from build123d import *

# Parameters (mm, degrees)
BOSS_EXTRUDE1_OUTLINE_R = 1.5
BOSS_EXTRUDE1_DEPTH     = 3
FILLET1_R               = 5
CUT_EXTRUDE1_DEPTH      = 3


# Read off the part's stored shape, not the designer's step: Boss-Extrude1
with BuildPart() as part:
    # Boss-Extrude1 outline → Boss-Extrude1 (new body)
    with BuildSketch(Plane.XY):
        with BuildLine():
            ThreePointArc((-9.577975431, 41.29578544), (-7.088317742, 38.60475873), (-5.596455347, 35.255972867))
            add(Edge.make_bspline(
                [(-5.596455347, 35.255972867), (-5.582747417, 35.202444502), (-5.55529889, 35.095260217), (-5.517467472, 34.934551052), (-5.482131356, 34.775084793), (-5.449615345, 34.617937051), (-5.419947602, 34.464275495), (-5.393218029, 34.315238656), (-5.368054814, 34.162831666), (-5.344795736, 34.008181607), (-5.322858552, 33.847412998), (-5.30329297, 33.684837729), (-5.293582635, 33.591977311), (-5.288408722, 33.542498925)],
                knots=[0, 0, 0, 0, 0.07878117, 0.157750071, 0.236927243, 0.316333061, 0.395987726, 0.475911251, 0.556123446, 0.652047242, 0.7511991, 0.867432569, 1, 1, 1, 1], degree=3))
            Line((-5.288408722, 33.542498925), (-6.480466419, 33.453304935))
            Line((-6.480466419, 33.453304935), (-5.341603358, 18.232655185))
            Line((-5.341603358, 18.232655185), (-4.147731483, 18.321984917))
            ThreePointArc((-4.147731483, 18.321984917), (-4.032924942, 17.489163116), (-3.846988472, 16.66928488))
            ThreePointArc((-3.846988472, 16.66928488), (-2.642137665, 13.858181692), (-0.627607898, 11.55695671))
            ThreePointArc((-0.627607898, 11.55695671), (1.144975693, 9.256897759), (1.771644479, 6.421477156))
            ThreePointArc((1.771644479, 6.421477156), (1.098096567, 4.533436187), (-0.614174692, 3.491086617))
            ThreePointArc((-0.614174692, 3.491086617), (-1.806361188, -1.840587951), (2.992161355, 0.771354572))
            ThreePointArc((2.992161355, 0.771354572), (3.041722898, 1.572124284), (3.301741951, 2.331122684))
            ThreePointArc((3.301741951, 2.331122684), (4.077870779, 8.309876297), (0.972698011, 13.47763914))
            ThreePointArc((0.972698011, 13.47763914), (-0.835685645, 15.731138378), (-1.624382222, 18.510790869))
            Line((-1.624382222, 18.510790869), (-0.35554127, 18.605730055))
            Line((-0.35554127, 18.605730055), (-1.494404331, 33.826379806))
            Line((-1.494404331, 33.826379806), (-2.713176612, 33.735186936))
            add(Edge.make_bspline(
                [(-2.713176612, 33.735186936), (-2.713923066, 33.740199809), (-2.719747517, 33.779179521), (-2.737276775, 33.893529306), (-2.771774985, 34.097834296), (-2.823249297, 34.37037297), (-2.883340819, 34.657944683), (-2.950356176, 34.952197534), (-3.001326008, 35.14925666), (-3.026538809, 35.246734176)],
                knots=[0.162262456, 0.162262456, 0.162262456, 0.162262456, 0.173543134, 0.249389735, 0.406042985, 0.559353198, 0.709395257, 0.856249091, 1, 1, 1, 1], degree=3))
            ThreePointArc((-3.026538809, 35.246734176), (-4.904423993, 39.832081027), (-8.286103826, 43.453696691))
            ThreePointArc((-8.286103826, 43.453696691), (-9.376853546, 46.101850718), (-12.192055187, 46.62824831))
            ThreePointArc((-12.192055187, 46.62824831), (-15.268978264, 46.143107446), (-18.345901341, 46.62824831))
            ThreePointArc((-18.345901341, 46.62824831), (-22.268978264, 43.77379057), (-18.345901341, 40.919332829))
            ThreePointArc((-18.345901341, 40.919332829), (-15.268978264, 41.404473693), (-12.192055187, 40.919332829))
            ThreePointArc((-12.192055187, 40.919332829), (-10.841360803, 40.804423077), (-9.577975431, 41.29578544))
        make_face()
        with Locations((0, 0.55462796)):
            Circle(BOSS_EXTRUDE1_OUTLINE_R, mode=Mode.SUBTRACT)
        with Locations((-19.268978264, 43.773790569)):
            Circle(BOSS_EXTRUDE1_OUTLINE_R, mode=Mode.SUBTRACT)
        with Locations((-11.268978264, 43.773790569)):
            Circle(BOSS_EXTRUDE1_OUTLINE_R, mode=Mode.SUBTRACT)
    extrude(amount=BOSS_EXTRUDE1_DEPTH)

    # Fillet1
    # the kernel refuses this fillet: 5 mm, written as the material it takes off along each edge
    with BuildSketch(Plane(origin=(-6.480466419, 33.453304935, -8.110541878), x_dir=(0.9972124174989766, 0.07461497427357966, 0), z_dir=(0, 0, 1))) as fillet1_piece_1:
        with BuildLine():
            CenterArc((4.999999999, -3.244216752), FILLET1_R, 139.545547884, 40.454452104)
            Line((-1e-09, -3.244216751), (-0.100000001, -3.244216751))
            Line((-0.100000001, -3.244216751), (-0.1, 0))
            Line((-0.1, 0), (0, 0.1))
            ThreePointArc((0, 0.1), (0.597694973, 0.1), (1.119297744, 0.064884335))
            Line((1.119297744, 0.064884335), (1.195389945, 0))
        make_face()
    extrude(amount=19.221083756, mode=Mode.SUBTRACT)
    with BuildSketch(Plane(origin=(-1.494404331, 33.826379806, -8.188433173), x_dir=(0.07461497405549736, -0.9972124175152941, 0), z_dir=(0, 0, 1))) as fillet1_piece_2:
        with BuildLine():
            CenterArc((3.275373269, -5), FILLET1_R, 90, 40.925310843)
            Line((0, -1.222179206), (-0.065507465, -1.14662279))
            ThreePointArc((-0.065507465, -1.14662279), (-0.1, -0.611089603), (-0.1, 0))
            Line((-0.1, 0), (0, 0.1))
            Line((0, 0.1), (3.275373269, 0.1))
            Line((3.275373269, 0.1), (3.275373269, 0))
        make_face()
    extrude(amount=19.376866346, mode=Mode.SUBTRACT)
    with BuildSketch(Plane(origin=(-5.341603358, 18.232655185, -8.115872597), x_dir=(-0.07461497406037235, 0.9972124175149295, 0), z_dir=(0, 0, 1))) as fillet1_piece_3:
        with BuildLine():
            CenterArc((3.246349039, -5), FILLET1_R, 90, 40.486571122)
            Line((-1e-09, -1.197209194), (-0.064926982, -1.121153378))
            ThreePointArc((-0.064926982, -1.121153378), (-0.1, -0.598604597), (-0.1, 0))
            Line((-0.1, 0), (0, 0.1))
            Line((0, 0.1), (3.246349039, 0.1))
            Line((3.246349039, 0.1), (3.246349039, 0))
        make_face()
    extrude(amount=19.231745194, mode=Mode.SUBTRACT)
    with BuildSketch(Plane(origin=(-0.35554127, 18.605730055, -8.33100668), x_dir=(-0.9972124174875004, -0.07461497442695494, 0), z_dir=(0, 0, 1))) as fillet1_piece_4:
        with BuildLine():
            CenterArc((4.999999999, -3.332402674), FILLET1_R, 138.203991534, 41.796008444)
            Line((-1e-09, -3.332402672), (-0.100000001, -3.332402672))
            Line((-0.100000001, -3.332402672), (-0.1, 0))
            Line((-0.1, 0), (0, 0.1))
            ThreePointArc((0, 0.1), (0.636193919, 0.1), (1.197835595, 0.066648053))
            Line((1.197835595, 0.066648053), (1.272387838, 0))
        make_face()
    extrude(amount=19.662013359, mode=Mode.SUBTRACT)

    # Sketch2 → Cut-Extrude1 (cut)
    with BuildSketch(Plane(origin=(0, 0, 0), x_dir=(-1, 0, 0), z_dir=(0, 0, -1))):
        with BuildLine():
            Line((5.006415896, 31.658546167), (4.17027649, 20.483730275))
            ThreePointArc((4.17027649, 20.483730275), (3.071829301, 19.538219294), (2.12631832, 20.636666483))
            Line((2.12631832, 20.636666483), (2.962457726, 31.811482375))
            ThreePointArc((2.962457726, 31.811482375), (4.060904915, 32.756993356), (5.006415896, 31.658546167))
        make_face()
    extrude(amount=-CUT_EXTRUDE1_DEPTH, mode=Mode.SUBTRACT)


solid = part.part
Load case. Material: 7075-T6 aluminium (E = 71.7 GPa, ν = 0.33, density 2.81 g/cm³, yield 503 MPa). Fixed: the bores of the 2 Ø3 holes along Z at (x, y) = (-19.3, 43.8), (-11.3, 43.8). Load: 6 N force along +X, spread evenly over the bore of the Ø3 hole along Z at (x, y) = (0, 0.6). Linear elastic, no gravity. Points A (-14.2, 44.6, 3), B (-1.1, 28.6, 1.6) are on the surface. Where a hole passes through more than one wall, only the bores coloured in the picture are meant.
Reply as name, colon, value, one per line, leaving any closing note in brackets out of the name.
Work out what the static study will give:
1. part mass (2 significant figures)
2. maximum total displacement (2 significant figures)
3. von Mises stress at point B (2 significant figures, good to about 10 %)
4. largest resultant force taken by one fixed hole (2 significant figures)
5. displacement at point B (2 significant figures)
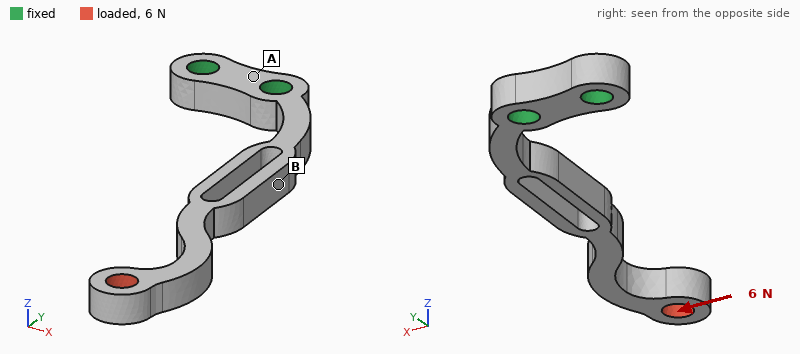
part mass: 1.6 g
maximum total displacement: 0.53 mm
von Mises stress at point B: 15 MPa
largest resultant force taken by one fixed hole: 5.8 N
displacement at point B: 0.12 mm
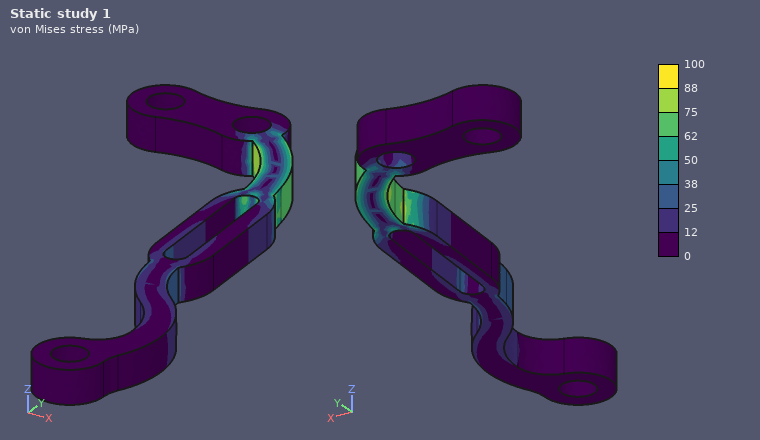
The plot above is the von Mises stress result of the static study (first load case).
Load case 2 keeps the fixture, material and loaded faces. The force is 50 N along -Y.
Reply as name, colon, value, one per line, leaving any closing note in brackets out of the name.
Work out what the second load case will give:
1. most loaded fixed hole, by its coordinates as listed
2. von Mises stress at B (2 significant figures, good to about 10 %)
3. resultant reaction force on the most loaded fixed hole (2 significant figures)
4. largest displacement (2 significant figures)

most loaded fixed hole, by its coordinates as listed: (-11.3, 43.8)
von Mises stress at B: 15 MPa
resultant reaction force on the most loaded fixed hole: 60 N
largest displacement: 0.61 mm
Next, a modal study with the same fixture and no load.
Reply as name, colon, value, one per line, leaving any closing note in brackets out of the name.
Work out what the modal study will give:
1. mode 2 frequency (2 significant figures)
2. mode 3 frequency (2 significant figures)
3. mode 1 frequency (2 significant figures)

mode 2 frequency: 880 Hz
mode 3 frequency: 5500 Hz
mode 1 frequency: 860 Hz
